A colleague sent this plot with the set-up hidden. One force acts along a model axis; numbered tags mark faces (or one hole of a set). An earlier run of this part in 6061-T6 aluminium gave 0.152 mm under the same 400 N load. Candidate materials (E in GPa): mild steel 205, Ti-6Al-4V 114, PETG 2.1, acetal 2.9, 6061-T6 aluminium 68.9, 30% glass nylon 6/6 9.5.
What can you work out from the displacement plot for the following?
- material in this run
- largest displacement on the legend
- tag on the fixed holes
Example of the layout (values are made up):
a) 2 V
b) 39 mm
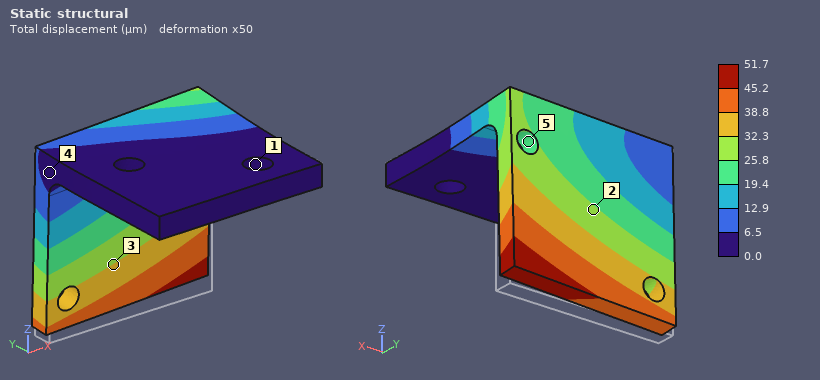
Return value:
a) mild steel
b) 51.7 µm
c) 1
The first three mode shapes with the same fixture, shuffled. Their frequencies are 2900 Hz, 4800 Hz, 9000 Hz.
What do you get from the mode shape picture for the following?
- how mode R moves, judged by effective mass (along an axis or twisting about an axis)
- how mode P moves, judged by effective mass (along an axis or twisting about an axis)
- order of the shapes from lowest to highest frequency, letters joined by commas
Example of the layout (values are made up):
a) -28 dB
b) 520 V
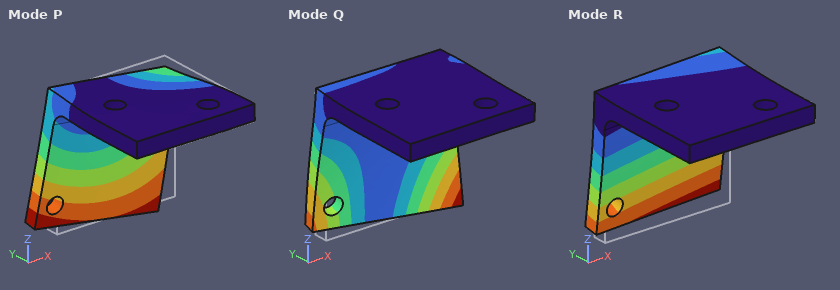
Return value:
a) along Y
b) along X
c) R, P, Q
